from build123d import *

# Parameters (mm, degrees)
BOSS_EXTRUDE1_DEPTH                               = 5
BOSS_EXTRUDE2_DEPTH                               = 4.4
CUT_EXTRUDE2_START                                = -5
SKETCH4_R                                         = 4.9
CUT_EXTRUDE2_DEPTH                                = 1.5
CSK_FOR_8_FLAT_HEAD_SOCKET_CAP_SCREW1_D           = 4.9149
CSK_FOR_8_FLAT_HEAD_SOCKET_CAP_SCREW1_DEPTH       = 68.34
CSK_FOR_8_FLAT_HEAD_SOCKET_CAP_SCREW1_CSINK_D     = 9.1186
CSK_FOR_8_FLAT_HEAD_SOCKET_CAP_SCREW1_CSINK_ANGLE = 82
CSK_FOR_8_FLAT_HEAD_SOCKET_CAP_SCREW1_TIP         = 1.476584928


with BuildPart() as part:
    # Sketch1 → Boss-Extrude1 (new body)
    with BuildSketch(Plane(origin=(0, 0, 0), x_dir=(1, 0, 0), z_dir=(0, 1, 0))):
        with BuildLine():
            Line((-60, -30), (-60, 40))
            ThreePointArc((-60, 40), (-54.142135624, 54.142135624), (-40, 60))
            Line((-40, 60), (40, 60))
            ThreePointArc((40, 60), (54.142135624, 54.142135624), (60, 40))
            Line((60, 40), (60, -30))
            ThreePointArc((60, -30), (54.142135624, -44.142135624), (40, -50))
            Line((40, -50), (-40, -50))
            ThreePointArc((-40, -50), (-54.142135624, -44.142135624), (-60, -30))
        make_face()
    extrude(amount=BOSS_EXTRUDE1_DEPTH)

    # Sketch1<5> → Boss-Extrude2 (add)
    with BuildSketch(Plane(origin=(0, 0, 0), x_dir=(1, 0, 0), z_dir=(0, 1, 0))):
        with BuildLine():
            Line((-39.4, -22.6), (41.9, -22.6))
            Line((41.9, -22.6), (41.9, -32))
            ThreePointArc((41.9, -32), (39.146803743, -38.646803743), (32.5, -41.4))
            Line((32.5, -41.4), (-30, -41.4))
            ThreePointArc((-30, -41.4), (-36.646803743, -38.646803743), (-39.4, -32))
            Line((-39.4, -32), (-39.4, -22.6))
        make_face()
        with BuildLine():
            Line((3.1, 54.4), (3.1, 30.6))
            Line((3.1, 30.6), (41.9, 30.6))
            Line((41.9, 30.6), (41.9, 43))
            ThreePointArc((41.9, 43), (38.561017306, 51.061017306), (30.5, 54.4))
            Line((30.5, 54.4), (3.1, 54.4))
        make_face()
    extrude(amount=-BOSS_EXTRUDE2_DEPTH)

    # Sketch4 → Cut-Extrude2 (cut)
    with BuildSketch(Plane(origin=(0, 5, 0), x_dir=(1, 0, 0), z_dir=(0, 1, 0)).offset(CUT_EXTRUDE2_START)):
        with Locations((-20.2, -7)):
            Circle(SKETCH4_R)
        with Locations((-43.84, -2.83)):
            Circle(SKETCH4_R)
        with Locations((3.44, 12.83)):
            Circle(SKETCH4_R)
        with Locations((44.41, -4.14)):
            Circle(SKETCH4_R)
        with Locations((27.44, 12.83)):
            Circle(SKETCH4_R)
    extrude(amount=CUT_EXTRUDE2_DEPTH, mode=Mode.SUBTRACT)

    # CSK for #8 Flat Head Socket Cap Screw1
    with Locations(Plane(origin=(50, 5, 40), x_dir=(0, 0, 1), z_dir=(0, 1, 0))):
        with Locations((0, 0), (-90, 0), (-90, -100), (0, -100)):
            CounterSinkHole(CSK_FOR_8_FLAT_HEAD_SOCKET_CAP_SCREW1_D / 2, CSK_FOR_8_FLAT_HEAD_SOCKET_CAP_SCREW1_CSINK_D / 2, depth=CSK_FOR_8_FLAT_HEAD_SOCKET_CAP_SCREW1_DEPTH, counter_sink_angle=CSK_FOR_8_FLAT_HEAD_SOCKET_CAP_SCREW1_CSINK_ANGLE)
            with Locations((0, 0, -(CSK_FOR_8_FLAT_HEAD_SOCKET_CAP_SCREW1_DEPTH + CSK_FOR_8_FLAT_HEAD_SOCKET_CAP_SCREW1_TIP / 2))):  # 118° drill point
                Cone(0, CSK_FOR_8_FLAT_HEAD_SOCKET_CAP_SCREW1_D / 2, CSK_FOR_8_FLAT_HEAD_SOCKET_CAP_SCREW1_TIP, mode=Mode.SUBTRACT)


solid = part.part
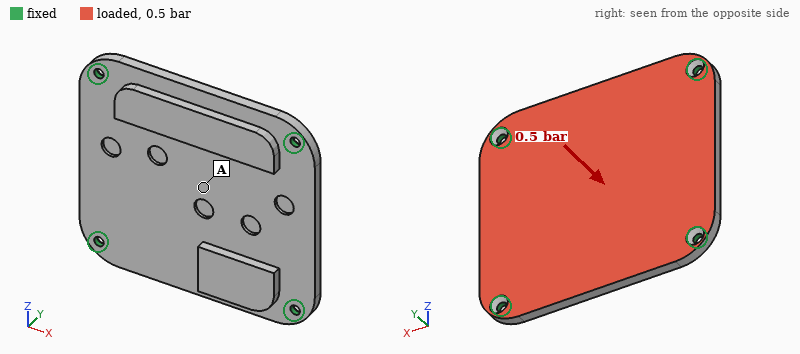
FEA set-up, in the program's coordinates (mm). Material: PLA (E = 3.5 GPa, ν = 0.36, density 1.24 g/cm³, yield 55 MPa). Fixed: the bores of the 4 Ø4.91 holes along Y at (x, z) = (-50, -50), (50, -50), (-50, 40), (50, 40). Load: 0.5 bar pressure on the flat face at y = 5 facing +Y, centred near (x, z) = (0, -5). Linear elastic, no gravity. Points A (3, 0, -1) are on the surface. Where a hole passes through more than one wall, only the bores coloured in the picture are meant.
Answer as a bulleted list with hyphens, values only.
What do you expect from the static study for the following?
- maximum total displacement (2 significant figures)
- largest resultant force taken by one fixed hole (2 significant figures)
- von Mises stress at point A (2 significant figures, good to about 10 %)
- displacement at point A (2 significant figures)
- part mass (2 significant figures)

- 0.84 mm
- 220 N
- 5.4 MPa
- 0.80 mm
- 91 g
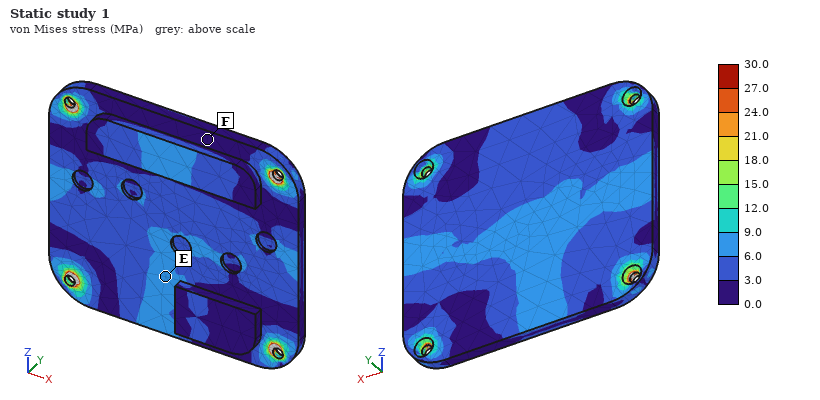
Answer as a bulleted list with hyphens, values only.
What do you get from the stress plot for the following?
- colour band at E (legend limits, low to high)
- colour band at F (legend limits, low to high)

- 6.0 to 9.0 MPa
- 0.0 to 3.0 MPa
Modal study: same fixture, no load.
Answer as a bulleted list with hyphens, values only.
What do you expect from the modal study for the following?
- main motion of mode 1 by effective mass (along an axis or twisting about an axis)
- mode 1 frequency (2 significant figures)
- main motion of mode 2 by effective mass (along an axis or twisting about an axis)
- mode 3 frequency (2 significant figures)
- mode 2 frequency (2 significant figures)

- along Y
- 580 Hz
- twisting about X
- 1100 Hz
- 920 Hz
